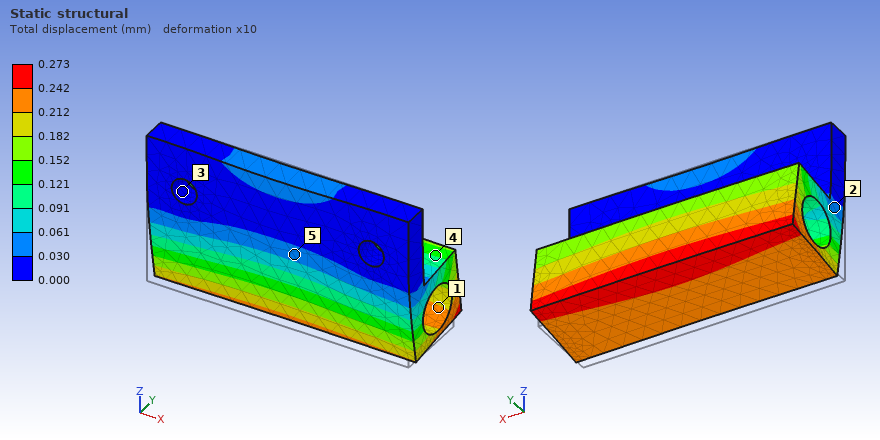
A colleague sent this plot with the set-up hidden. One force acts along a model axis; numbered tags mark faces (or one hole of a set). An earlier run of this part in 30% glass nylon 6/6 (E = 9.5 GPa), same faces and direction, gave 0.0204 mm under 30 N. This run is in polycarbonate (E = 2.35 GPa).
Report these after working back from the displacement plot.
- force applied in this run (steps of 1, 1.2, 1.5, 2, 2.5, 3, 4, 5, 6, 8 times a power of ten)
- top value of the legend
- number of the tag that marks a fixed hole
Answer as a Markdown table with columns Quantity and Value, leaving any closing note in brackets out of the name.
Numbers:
| Quantity | Value |
|---|---|
| force applied in this run | 100 N |
| top value of the legend | 0.273 mm |
| number of the tag that marks a fixed hole | 3 |
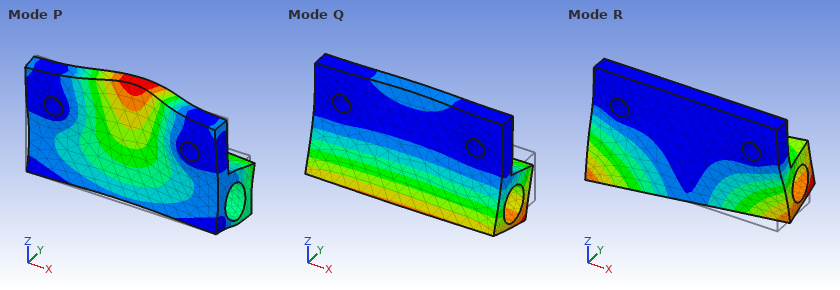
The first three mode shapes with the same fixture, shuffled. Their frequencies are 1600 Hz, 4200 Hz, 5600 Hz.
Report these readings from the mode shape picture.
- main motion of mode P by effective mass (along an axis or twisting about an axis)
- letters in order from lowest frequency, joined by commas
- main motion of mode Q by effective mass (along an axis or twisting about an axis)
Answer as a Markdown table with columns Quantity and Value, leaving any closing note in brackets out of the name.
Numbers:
| Quantity | Value |
|---|---|
| main motion of mode P by effective mass | along Y |
| letters in order from lowest frequency, joined by commas | Q, R, P |
| main motion of mode Q by effective mass | along Y |
